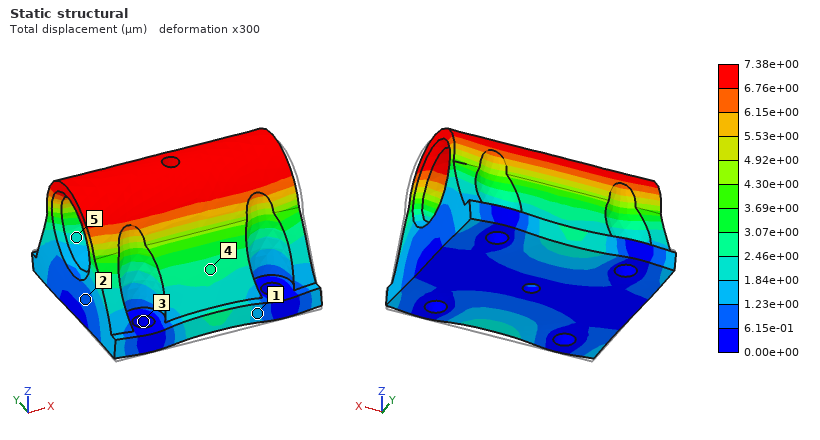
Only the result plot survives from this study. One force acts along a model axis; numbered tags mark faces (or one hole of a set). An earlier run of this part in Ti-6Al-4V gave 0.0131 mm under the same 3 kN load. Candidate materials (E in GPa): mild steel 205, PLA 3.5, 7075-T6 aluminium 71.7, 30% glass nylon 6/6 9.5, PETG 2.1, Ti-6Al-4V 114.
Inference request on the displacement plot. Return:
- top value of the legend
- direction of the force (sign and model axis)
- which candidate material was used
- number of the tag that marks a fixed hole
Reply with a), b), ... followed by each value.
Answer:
a) 7.38e+00 µm
b) +Y
c) mild steel
d) 3
